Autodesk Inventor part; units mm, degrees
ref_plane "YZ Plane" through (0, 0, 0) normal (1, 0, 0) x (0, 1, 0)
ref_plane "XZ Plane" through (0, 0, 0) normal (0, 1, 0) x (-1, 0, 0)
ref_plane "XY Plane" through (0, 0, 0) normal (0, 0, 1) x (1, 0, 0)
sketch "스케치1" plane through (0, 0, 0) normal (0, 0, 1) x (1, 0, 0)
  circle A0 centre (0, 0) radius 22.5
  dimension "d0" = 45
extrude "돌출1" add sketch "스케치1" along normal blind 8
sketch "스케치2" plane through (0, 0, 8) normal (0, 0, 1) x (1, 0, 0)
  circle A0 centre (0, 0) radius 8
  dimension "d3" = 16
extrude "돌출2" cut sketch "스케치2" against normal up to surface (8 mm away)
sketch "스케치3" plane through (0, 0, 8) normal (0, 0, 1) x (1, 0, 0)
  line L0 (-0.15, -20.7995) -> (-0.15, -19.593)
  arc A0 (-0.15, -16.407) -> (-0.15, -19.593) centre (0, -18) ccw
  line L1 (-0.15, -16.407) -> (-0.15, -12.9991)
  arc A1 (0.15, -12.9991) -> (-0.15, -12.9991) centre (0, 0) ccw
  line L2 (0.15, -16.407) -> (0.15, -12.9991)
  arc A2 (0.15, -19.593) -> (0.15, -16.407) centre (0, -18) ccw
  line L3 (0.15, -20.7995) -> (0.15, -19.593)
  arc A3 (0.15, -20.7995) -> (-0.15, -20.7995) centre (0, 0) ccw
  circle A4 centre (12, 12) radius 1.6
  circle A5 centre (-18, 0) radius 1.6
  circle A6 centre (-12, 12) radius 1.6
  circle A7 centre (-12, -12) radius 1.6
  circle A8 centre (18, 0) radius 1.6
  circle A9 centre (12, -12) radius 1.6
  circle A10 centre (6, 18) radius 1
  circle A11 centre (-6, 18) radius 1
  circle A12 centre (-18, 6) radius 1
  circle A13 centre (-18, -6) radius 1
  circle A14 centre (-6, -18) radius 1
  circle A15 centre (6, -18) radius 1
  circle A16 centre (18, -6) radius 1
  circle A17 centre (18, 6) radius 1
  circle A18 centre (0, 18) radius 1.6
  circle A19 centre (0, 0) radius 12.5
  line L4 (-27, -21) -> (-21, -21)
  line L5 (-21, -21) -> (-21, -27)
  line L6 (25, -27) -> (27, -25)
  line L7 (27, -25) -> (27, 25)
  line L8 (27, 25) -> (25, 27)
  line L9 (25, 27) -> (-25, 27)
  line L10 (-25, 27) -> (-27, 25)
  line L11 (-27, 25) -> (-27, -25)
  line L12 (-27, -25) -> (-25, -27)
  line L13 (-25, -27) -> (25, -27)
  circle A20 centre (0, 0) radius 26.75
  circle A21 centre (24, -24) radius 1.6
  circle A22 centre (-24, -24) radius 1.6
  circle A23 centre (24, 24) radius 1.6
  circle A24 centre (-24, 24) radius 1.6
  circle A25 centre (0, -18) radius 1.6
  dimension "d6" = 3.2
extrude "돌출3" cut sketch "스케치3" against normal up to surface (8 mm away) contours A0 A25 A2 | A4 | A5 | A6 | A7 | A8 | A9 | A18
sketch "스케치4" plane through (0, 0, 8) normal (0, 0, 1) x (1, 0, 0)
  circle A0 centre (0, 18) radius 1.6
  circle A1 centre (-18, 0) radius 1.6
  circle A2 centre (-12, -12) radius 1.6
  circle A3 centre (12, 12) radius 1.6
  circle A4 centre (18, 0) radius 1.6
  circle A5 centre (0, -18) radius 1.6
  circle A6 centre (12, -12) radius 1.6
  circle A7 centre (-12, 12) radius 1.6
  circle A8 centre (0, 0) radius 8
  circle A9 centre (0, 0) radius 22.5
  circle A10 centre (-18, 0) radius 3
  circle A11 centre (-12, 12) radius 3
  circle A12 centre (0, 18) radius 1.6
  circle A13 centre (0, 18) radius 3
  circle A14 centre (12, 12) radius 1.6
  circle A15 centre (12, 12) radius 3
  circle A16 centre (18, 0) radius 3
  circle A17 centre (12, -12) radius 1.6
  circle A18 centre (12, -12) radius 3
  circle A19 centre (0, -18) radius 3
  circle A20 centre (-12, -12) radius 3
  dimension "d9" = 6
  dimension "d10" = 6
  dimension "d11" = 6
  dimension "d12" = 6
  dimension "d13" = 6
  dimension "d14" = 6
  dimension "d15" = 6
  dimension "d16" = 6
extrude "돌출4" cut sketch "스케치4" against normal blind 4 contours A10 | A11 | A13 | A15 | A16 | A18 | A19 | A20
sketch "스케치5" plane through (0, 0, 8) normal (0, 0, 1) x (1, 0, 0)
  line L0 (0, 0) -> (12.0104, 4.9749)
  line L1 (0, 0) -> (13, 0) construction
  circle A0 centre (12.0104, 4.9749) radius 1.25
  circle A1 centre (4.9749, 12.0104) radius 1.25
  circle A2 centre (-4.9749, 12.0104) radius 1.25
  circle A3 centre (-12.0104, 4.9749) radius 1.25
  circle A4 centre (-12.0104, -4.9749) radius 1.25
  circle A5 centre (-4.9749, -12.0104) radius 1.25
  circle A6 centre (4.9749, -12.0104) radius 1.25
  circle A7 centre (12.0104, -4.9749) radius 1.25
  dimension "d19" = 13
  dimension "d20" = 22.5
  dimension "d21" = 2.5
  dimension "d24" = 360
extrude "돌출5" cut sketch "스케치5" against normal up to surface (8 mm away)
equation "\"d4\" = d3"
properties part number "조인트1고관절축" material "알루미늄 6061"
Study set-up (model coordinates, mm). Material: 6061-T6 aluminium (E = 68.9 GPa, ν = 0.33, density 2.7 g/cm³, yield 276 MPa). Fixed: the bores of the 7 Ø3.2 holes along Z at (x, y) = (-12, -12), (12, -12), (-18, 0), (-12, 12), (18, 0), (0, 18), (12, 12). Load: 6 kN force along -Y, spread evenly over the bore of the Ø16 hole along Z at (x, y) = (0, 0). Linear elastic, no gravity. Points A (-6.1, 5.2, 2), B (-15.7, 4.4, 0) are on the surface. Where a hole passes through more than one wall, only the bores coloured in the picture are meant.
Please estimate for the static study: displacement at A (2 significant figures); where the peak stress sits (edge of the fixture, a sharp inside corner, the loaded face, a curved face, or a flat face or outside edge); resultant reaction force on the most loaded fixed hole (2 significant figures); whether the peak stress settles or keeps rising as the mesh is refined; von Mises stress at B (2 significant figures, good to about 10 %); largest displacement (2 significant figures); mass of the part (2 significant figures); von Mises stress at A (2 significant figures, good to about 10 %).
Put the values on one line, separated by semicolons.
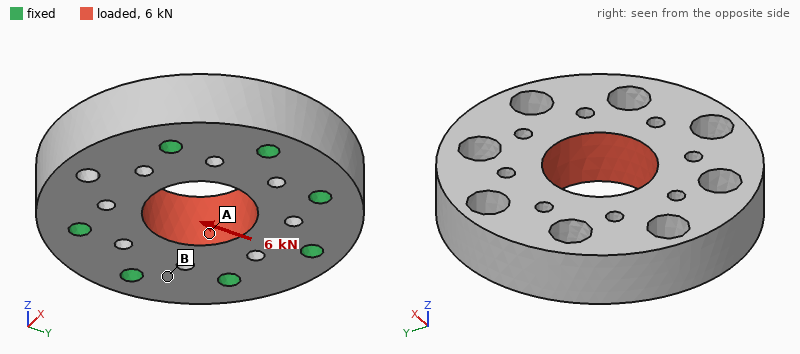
3.6 µm; edge of the fixture; 1.2 kN; keeps rising; 9.8 MPa; 7.7 µm; 26 g; 22 MPa
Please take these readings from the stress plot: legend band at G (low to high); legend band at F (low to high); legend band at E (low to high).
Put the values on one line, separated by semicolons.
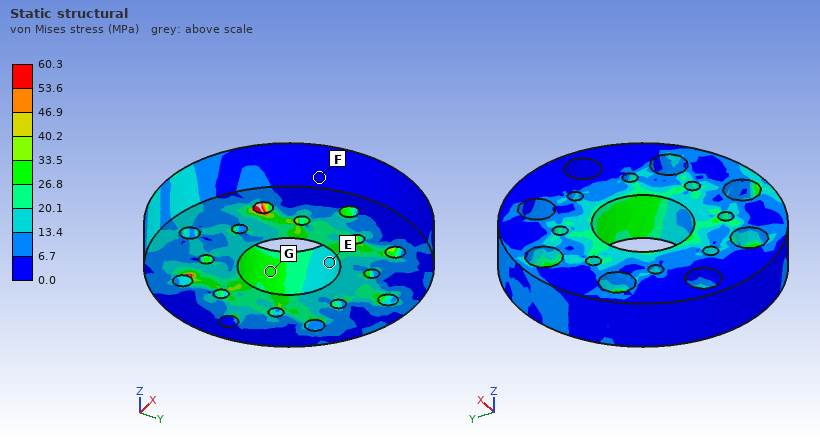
26.8 to 33.5 MPa; 0.0 to 6.7 MPa; 13.4 to 20.1 MPa
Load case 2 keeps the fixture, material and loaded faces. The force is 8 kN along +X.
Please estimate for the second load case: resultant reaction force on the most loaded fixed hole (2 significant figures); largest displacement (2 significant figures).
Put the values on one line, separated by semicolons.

1.4 kN; 7.2 µm
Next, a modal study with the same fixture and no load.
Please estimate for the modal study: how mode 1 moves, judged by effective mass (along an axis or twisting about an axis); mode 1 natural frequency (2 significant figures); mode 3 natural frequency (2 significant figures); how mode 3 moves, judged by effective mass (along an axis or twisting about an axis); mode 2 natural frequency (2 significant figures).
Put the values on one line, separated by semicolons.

along Z; 27 kHz; 46 kHz; along Y; 38 kHz
